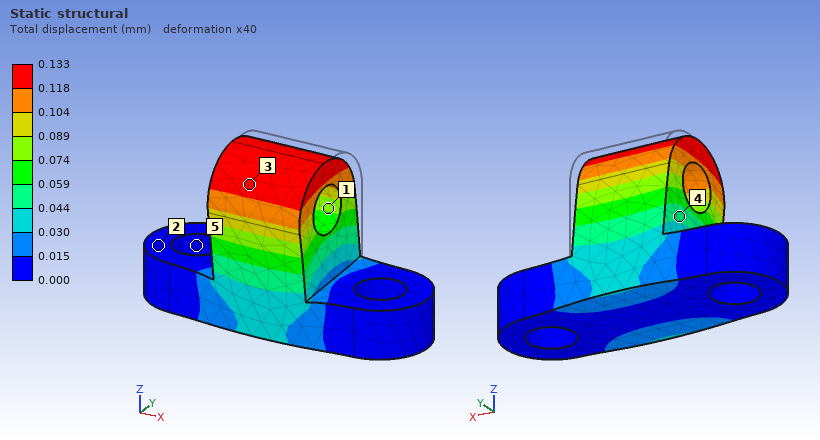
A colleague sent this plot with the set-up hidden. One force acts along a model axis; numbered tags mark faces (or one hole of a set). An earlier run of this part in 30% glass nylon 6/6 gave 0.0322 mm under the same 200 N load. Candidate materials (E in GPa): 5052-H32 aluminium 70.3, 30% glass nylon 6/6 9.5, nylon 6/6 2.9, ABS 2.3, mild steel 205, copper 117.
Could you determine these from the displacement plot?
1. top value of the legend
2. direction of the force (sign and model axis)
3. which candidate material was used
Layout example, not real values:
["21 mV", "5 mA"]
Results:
["0.133 mm", "-Y", "ABS"]
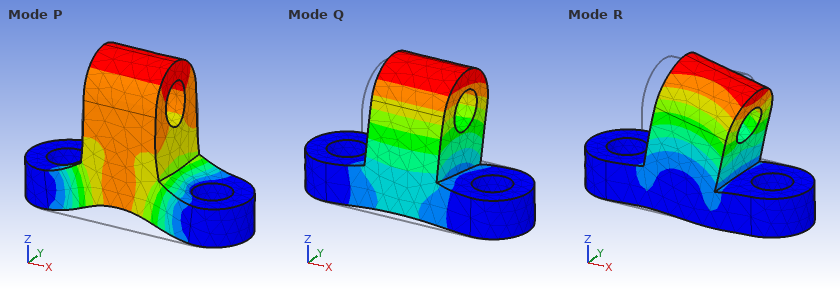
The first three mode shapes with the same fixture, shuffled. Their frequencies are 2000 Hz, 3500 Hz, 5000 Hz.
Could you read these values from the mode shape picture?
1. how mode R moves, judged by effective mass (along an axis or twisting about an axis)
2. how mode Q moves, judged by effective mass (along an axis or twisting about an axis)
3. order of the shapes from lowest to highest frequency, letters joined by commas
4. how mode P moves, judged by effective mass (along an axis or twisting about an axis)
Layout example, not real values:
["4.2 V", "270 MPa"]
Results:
["along X", "along Y", "Q, R, P", "along Z"]
